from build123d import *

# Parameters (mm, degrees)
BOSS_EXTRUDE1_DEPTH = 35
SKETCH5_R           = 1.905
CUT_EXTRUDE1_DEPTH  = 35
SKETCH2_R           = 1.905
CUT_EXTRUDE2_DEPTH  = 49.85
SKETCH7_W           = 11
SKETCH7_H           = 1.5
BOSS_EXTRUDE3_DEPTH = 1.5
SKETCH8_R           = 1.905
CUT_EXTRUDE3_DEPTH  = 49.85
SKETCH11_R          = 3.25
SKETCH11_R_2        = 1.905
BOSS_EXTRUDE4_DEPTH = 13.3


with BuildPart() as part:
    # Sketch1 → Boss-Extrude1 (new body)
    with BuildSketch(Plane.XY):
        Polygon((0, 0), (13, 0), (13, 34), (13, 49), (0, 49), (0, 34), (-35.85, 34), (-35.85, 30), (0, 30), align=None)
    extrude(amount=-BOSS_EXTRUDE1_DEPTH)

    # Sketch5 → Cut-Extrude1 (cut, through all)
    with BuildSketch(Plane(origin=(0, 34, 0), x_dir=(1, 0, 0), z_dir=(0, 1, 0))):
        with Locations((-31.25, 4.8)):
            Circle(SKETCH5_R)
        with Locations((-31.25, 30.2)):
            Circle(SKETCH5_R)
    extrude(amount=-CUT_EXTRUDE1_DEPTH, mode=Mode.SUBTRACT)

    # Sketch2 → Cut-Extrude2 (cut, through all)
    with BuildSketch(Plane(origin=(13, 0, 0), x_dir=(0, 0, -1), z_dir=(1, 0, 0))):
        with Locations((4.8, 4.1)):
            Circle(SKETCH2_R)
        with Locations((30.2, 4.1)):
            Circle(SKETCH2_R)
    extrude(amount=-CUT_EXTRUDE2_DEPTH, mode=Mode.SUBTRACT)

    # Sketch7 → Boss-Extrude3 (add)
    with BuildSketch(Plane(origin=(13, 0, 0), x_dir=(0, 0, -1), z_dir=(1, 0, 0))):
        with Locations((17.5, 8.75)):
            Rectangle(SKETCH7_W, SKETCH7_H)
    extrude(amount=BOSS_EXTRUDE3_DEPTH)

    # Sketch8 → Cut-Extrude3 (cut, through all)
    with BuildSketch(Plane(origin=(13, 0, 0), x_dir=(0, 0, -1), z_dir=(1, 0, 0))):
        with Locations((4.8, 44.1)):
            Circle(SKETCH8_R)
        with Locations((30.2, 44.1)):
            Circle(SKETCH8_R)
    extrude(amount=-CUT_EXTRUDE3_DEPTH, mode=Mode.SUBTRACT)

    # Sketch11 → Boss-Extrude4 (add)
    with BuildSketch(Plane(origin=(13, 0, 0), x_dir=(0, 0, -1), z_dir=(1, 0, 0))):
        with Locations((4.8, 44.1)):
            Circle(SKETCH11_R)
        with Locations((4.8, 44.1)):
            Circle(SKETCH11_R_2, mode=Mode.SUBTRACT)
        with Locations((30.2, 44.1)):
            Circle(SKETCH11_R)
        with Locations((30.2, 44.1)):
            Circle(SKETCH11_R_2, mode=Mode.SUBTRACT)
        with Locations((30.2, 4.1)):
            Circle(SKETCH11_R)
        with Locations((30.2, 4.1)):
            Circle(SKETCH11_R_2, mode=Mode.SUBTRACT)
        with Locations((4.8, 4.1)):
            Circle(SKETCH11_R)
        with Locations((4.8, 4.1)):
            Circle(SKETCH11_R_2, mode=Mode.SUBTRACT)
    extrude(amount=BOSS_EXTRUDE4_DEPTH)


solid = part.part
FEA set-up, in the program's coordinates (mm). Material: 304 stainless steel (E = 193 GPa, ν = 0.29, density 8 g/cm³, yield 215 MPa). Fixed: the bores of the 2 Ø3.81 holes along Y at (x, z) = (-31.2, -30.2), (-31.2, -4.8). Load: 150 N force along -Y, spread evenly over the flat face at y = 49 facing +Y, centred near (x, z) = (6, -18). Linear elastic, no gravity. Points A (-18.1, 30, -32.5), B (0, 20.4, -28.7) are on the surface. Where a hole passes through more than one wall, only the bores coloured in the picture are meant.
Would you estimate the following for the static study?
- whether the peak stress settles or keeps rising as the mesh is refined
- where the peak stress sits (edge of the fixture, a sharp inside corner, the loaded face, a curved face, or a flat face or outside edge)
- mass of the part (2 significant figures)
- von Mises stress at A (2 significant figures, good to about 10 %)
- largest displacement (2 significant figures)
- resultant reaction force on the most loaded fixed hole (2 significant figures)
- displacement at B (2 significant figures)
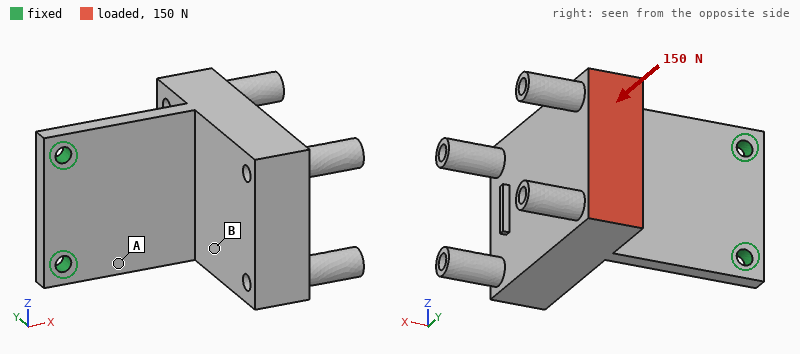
keeps rising
edge of the fixture
220 g
41 MPa
0.16 mm
75 N
0.068 mm
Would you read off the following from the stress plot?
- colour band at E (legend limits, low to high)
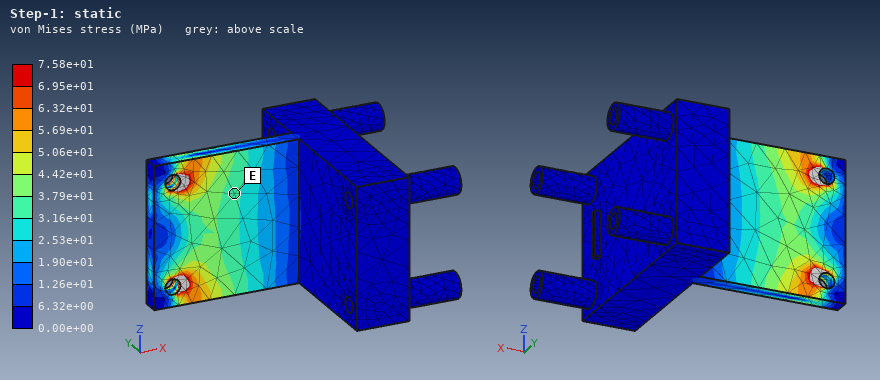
3.16e+01 to 3.79e+01 MPa
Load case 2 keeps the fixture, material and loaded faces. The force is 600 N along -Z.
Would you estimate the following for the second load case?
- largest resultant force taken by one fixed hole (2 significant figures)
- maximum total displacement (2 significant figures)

970 N
0.11 mm
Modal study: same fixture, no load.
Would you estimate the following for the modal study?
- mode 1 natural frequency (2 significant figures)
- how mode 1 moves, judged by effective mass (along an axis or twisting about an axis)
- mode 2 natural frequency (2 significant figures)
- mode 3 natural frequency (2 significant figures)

420 Hz
along Y
1100 Hz
2100 Hz
